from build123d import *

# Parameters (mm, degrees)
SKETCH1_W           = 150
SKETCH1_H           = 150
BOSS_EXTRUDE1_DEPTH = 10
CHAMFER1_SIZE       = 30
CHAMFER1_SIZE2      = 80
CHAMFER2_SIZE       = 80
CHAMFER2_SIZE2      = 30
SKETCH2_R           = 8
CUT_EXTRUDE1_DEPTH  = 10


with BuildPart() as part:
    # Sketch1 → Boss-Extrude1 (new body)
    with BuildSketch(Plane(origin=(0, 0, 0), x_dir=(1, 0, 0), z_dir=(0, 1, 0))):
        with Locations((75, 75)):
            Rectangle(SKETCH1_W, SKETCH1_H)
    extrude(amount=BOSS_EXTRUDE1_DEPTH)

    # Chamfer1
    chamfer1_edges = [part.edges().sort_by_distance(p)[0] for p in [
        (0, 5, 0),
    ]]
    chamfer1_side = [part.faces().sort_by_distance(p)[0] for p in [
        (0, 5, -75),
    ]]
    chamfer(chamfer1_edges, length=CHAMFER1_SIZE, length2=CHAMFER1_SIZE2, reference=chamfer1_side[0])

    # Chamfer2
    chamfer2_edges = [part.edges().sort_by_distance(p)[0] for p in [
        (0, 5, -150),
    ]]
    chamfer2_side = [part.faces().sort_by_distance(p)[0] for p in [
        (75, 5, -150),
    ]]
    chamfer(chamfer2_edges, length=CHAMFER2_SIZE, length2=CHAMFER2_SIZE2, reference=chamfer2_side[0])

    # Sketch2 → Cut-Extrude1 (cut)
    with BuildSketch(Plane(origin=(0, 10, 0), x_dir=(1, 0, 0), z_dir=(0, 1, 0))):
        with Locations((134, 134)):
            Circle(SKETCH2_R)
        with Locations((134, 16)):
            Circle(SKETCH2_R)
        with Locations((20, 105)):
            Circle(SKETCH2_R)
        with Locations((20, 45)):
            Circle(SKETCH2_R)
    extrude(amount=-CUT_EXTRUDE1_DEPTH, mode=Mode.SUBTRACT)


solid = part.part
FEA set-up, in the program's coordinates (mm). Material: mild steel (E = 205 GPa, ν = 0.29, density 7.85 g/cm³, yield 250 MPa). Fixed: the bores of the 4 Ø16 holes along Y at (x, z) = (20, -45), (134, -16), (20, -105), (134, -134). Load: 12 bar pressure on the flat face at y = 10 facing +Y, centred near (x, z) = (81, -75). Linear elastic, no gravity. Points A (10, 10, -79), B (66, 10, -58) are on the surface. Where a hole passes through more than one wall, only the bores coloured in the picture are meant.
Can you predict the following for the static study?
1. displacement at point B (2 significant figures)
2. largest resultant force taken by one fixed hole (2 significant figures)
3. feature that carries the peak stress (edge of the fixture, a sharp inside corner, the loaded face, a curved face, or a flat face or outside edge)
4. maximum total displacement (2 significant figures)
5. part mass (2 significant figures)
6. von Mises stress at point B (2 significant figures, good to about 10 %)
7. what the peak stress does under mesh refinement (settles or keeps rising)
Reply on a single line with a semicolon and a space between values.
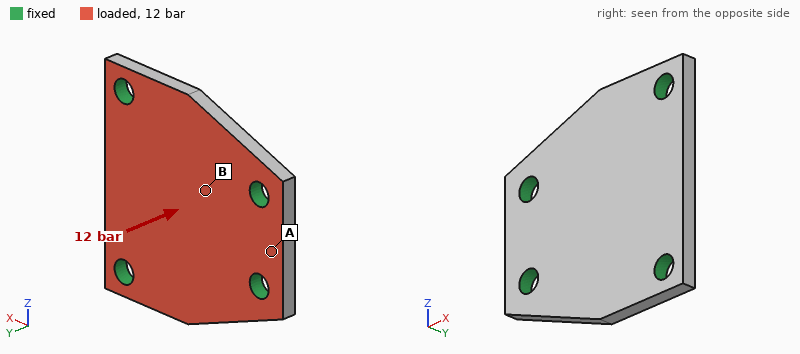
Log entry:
35 µm; 6.1 kN; edge of the fixture; 46 µm; 1.5 kg; 26 MPa; keeps rising
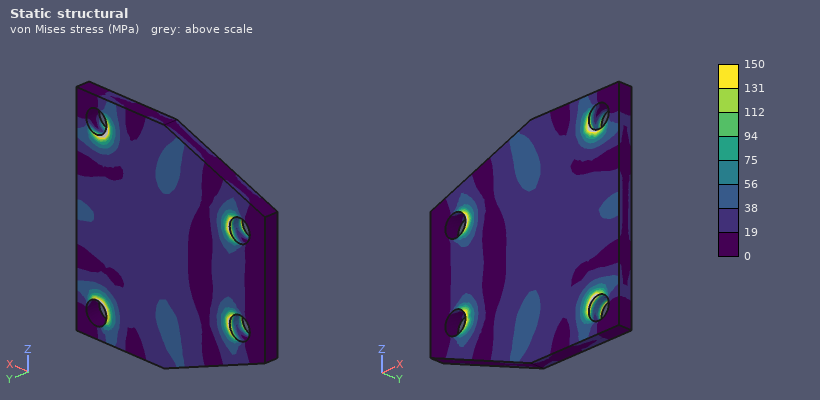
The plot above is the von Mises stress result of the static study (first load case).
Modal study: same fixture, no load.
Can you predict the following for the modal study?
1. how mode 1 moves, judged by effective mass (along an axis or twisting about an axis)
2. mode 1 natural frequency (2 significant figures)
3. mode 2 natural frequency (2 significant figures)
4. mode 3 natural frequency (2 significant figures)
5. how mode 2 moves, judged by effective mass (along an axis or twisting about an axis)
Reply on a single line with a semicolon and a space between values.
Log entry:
along Y; 3500 Hz; 4300 Hz; 4500 Hz; twisting about X
